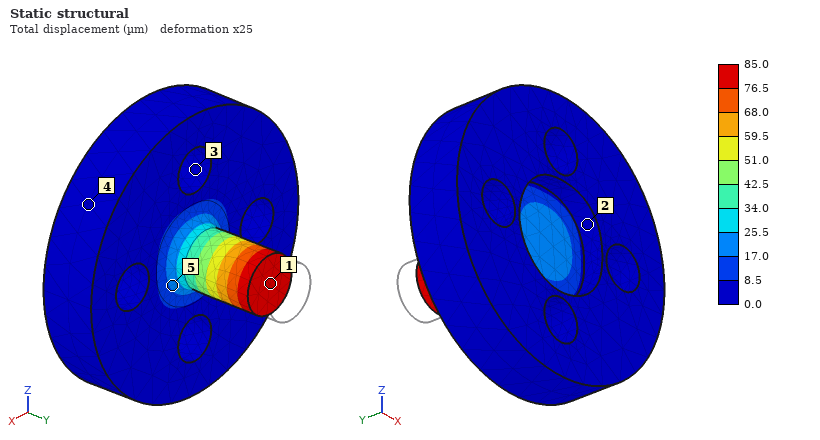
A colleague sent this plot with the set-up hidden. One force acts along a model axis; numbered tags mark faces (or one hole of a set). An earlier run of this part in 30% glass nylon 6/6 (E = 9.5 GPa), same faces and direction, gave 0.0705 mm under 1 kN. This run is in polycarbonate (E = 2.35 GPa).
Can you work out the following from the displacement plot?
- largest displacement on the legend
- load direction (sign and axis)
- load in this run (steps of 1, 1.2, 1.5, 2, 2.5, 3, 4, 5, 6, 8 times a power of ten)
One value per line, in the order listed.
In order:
85.0 µm
-Y
300 N
